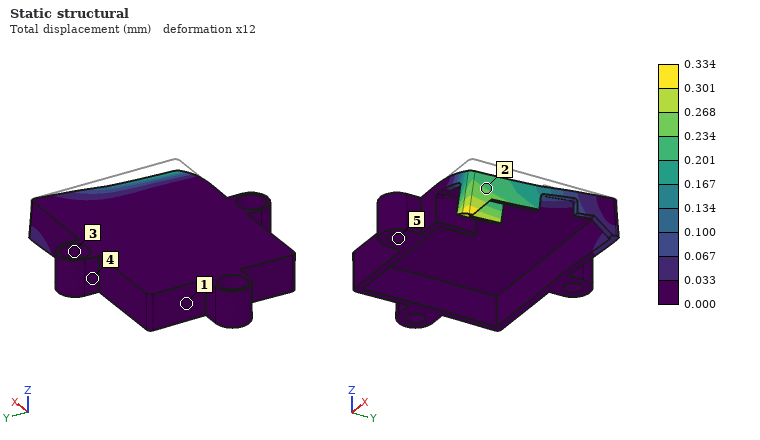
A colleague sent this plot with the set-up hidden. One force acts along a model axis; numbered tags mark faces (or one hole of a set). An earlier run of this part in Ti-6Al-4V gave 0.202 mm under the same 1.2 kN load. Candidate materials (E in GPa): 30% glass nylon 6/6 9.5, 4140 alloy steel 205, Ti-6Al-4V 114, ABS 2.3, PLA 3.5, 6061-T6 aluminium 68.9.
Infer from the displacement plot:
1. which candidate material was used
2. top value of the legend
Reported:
6061-T6 aluminium
0.334 mm
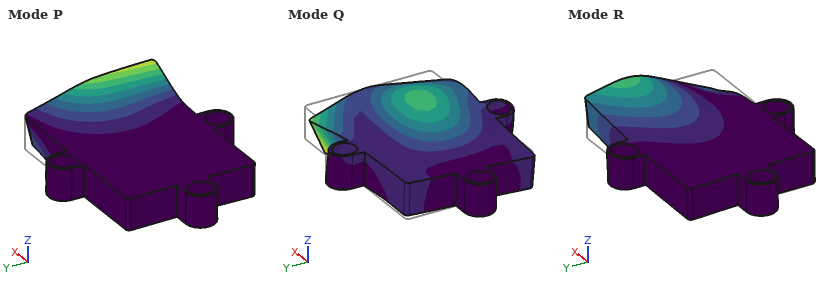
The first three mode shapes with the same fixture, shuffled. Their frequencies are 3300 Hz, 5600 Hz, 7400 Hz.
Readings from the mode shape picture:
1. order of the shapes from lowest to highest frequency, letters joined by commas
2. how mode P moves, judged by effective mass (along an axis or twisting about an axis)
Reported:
P, R, Q
along Z
